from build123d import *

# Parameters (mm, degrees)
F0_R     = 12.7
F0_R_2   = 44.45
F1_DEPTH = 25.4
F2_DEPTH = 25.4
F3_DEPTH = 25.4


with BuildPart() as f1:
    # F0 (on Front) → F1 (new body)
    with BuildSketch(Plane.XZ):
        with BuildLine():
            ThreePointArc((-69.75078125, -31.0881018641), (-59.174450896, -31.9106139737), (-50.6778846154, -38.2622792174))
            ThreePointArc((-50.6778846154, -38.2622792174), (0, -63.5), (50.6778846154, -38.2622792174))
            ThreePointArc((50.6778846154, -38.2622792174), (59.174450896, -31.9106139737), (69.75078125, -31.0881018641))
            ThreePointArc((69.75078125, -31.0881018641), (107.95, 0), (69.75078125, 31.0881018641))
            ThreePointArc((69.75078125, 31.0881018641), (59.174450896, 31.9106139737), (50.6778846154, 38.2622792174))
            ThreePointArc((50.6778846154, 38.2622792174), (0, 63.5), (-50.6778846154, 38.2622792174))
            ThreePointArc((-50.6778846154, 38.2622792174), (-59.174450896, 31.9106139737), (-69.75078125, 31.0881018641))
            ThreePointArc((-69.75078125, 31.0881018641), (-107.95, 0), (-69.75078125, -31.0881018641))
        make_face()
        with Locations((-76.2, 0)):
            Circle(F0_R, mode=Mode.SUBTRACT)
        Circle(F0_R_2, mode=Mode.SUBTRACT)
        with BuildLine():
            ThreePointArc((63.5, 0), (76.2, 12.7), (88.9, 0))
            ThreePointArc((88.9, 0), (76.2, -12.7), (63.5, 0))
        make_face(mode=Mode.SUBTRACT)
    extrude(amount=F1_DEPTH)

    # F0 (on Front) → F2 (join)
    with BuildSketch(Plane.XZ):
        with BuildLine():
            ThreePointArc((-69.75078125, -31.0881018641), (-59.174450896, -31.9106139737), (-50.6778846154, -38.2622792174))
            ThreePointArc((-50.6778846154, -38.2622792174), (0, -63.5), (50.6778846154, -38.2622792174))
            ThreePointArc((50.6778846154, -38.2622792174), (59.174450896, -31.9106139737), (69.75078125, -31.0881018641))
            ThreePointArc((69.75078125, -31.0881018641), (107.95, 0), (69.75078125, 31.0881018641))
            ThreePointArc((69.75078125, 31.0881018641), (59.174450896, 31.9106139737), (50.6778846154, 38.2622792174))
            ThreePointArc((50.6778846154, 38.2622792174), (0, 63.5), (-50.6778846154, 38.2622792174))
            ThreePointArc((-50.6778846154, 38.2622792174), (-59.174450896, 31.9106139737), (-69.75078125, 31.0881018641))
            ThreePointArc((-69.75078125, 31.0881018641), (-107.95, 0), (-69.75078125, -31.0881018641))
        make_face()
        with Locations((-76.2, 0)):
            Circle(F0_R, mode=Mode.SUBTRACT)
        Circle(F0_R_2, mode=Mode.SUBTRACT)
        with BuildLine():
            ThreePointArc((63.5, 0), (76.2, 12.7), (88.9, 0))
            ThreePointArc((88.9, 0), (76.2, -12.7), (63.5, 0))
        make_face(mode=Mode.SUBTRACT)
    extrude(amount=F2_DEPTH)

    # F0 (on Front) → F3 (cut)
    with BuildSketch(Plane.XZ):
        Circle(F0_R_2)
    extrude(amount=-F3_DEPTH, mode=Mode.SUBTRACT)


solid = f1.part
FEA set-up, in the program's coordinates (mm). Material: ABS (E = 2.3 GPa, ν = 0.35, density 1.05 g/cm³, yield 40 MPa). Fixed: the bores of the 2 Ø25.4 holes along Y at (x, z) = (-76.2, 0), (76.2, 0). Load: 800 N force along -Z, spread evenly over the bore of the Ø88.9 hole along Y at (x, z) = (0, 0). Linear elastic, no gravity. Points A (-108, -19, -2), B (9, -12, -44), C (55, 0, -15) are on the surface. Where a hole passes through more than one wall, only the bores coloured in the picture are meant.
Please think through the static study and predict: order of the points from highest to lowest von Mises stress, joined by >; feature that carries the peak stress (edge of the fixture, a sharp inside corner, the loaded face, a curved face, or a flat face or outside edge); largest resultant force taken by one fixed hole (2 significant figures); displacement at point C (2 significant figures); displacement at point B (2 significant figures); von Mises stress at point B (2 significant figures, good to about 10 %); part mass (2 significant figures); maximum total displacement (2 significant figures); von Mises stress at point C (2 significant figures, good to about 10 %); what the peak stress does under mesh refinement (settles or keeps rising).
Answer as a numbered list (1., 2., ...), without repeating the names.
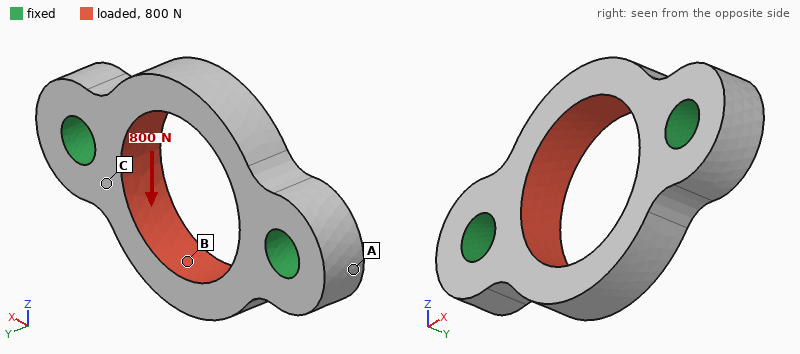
1. C > B > A
2. edge of the fixture
3. 400 N
4. 5.0 µm
5. 18 µm
6. 0.23 MPa
7. 280 g
8. 19 µm
9. 0.46 MPa
10. keeps rising
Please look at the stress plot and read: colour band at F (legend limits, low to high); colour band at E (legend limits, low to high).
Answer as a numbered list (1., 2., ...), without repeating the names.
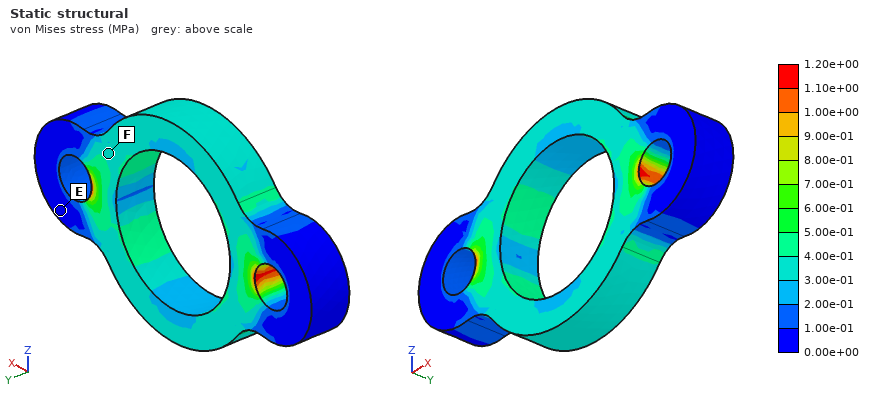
1. 3.00e-01 to 4.00e-01 MPa
2. 0.00e+00 to 1.00e-01 MPa
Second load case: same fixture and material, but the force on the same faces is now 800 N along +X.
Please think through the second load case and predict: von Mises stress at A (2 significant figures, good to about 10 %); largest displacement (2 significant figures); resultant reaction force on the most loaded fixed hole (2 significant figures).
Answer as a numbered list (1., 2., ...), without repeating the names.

1. 0.091 MPa
2. 17 µm
3. 400 N
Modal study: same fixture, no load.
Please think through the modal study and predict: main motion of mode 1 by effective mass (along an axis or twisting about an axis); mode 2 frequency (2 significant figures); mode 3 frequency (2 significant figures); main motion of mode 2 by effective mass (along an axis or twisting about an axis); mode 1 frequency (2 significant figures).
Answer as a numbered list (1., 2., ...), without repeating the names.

1. twisting about X
2. 1200 Hz
3. 2400 Hz
4. along Y
5. 1100 Hz
